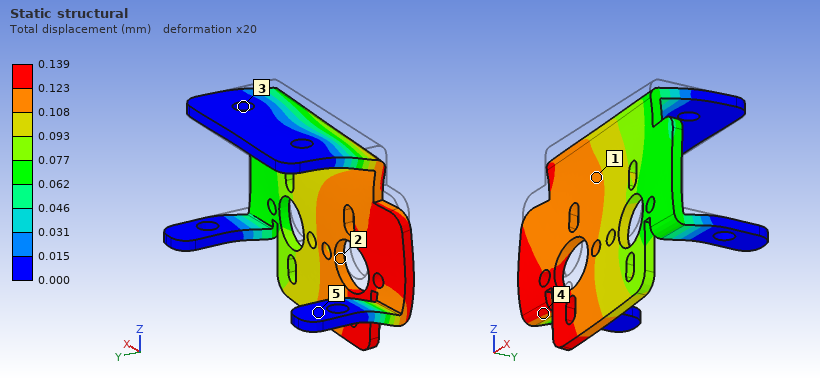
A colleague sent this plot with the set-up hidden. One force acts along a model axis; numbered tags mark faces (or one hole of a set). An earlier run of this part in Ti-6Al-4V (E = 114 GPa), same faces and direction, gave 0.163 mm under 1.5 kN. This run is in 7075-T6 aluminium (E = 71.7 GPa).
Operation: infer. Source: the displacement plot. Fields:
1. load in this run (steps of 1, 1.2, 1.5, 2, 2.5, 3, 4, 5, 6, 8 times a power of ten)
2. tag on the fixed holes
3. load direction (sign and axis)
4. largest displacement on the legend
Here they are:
800 N
3
-Z
0.139 mm
